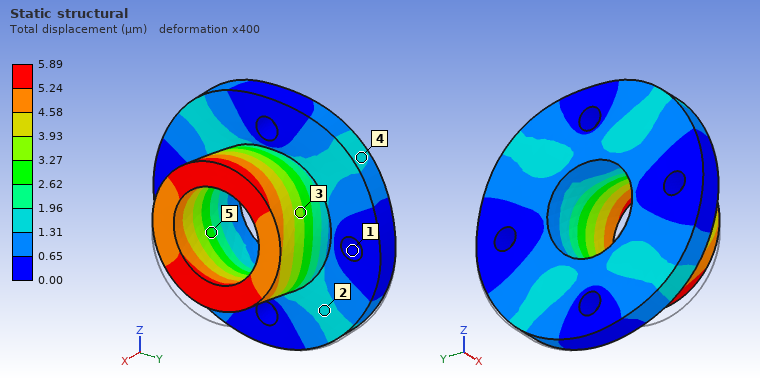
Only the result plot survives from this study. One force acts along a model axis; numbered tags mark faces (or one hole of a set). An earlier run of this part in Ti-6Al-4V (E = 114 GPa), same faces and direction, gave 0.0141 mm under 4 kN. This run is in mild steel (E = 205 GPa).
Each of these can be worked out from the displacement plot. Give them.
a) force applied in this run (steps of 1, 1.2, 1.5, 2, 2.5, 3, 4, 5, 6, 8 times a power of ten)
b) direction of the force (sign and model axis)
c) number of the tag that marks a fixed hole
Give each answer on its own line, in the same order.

3 kN
+Z
1
